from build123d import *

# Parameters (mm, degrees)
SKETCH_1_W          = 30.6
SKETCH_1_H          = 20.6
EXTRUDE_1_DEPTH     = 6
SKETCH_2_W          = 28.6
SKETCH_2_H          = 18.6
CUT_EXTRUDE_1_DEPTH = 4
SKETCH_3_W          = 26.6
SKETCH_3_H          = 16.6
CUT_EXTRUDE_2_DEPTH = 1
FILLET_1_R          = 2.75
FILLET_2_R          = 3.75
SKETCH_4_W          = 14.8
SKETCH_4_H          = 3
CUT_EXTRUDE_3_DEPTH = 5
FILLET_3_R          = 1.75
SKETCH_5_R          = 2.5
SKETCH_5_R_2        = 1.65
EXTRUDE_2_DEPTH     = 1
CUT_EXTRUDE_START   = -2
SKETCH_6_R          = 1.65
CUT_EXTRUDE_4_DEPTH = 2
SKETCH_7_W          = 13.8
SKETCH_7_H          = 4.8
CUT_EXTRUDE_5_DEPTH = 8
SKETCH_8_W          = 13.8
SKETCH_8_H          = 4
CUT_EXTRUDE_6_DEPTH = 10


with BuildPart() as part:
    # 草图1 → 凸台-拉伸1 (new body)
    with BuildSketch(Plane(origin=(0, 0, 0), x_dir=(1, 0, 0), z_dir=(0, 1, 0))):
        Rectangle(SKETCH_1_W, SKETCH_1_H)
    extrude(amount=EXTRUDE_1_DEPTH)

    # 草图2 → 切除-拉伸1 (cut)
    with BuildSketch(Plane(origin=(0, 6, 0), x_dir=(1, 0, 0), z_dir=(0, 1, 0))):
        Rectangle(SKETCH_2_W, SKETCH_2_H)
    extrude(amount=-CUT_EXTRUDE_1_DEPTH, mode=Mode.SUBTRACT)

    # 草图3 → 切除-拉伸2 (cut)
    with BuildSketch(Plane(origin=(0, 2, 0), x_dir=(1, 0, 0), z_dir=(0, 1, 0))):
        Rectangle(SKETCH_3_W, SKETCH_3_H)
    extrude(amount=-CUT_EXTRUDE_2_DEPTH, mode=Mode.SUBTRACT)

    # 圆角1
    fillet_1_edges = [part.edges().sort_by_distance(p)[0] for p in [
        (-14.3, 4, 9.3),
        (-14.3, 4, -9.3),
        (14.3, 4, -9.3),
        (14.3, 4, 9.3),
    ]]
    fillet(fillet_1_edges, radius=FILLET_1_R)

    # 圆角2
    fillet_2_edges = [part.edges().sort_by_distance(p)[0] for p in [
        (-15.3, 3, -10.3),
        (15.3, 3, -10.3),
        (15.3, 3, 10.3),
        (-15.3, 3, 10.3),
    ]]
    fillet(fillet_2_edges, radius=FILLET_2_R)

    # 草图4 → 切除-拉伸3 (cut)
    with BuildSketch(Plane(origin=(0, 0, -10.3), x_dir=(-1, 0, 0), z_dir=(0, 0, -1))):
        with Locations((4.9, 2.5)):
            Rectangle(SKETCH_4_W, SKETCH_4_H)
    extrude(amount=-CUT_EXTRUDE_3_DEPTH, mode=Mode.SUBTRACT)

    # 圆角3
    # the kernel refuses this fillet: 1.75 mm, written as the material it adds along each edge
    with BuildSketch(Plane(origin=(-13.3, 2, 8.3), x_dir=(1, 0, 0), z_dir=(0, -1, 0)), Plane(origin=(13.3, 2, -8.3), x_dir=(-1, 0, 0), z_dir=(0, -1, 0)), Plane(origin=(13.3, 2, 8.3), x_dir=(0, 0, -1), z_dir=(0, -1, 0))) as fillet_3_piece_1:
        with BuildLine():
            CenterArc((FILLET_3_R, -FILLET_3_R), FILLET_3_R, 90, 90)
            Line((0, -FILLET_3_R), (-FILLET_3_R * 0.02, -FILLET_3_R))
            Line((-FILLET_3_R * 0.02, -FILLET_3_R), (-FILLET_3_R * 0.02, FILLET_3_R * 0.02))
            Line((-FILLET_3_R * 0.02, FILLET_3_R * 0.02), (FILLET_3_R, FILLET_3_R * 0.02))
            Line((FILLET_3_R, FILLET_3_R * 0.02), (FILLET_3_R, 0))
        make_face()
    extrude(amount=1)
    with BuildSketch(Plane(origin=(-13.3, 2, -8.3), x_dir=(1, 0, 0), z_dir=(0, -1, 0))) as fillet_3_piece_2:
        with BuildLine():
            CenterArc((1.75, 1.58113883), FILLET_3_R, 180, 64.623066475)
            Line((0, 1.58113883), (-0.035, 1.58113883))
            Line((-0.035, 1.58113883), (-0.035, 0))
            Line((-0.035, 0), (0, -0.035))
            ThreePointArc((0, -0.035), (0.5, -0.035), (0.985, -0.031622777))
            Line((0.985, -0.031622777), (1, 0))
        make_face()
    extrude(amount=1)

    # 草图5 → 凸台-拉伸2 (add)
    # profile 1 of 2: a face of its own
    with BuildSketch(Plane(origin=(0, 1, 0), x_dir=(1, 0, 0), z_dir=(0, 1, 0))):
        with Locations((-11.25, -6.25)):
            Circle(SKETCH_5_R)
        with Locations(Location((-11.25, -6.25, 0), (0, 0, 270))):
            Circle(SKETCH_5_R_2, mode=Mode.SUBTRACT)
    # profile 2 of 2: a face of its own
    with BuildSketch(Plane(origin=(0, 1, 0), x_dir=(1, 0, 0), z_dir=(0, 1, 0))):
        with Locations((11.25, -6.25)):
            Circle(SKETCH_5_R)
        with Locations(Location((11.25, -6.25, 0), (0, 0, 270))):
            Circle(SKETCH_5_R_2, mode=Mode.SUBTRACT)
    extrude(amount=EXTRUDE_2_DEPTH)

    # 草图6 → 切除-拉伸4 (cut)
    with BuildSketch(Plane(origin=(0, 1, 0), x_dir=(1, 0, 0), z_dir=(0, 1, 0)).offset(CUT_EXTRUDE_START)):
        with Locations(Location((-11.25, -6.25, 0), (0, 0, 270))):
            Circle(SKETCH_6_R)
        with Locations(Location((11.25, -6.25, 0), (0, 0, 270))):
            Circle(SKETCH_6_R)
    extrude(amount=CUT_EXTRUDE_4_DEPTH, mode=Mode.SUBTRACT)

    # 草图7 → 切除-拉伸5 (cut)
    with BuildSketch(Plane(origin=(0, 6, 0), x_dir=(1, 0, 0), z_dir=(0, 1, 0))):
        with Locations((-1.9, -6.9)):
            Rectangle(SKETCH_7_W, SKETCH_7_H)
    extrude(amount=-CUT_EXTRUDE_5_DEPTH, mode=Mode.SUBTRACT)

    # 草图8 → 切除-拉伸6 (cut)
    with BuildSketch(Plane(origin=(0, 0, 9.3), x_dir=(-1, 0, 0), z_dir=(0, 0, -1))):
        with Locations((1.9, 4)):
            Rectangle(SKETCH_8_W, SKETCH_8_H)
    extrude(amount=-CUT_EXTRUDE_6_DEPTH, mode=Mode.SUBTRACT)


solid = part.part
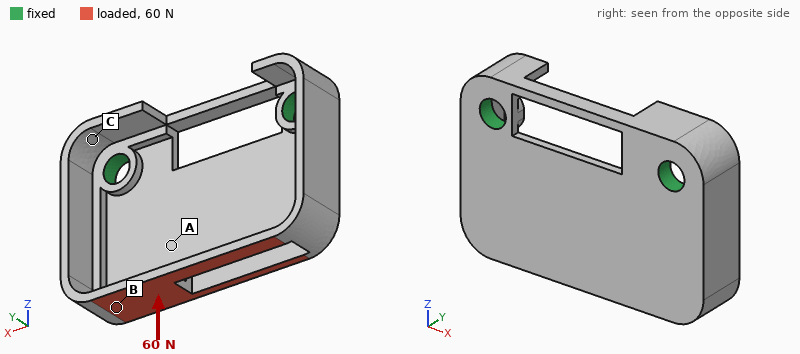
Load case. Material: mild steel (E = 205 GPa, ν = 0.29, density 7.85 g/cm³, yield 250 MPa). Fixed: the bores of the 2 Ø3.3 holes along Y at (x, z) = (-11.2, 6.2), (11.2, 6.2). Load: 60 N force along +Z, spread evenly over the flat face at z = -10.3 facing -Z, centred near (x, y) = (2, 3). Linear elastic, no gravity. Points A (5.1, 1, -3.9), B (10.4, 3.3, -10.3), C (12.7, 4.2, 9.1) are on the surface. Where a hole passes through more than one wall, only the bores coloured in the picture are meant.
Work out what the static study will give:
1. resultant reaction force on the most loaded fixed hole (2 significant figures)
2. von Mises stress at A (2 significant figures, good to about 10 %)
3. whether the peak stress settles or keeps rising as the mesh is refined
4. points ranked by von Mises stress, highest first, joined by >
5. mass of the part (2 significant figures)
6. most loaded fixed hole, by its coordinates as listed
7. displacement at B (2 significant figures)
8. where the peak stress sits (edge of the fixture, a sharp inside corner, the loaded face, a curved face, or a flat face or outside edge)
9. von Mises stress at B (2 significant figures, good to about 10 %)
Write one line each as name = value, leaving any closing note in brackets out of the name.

resultant reaction force on the most loaded fixed hole = 38 N
von Mises stress at A = 12 MPa
whether the peak stress settles or keeps rising as the mesh is refined = keeps rising
points ranked by von Mises stress, highest first, joined by > = B > A > C
mass of the part = 7.7 g
most loaded fixed hole, by its coordinates as listed = (11.2, 6.2)
displacement at B = 5.2 µm
where the peak stress sits = a sharp inside corner
von Mises stress at B = 26 MPa
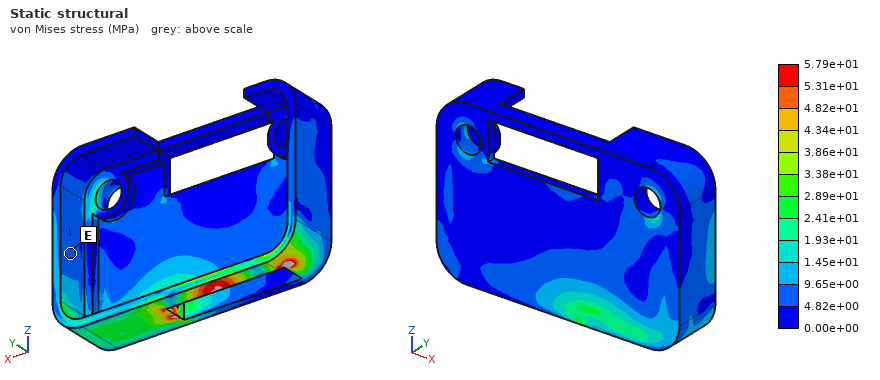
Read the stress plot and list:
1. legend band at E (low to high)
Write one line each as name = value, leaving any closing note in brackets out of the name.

legend band at E = 4.82e+00 to 9.65e+00 MPa
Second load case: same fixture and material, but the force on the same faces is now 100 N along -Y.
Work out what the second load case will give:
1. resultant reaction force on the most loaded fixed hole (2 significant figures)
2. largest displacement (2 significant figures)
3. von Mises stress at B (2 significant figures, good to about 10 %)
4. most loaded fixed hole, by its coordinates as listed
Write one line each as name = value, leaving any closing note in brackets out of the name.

resultant reaction force on the most loaded fixed hole = 68 N
largest displacement = 53 µm
von Mises stress at B = 43 MPa
most loaded fixed hole, by its coordinates as listed = (11.2, 6.2)
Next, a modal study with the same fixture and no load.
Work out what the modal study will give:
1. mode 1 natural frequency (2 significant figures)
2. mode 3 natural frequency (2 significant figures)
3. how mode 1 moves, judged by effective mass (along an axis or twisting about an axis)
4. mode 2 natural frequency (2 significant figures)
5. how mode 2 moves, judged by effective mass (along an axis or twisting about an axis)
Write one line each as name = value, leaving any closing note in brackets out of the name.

mode 1 natural frequency = 5700 Hz
mode 3 natural frequency = 12 kHz
how mode 1 moves, judged by effective mass = along Y
mode 2 natural frequency = 8800 Hz
how mode 2 moves, judged by effective mass = twisting about Z
